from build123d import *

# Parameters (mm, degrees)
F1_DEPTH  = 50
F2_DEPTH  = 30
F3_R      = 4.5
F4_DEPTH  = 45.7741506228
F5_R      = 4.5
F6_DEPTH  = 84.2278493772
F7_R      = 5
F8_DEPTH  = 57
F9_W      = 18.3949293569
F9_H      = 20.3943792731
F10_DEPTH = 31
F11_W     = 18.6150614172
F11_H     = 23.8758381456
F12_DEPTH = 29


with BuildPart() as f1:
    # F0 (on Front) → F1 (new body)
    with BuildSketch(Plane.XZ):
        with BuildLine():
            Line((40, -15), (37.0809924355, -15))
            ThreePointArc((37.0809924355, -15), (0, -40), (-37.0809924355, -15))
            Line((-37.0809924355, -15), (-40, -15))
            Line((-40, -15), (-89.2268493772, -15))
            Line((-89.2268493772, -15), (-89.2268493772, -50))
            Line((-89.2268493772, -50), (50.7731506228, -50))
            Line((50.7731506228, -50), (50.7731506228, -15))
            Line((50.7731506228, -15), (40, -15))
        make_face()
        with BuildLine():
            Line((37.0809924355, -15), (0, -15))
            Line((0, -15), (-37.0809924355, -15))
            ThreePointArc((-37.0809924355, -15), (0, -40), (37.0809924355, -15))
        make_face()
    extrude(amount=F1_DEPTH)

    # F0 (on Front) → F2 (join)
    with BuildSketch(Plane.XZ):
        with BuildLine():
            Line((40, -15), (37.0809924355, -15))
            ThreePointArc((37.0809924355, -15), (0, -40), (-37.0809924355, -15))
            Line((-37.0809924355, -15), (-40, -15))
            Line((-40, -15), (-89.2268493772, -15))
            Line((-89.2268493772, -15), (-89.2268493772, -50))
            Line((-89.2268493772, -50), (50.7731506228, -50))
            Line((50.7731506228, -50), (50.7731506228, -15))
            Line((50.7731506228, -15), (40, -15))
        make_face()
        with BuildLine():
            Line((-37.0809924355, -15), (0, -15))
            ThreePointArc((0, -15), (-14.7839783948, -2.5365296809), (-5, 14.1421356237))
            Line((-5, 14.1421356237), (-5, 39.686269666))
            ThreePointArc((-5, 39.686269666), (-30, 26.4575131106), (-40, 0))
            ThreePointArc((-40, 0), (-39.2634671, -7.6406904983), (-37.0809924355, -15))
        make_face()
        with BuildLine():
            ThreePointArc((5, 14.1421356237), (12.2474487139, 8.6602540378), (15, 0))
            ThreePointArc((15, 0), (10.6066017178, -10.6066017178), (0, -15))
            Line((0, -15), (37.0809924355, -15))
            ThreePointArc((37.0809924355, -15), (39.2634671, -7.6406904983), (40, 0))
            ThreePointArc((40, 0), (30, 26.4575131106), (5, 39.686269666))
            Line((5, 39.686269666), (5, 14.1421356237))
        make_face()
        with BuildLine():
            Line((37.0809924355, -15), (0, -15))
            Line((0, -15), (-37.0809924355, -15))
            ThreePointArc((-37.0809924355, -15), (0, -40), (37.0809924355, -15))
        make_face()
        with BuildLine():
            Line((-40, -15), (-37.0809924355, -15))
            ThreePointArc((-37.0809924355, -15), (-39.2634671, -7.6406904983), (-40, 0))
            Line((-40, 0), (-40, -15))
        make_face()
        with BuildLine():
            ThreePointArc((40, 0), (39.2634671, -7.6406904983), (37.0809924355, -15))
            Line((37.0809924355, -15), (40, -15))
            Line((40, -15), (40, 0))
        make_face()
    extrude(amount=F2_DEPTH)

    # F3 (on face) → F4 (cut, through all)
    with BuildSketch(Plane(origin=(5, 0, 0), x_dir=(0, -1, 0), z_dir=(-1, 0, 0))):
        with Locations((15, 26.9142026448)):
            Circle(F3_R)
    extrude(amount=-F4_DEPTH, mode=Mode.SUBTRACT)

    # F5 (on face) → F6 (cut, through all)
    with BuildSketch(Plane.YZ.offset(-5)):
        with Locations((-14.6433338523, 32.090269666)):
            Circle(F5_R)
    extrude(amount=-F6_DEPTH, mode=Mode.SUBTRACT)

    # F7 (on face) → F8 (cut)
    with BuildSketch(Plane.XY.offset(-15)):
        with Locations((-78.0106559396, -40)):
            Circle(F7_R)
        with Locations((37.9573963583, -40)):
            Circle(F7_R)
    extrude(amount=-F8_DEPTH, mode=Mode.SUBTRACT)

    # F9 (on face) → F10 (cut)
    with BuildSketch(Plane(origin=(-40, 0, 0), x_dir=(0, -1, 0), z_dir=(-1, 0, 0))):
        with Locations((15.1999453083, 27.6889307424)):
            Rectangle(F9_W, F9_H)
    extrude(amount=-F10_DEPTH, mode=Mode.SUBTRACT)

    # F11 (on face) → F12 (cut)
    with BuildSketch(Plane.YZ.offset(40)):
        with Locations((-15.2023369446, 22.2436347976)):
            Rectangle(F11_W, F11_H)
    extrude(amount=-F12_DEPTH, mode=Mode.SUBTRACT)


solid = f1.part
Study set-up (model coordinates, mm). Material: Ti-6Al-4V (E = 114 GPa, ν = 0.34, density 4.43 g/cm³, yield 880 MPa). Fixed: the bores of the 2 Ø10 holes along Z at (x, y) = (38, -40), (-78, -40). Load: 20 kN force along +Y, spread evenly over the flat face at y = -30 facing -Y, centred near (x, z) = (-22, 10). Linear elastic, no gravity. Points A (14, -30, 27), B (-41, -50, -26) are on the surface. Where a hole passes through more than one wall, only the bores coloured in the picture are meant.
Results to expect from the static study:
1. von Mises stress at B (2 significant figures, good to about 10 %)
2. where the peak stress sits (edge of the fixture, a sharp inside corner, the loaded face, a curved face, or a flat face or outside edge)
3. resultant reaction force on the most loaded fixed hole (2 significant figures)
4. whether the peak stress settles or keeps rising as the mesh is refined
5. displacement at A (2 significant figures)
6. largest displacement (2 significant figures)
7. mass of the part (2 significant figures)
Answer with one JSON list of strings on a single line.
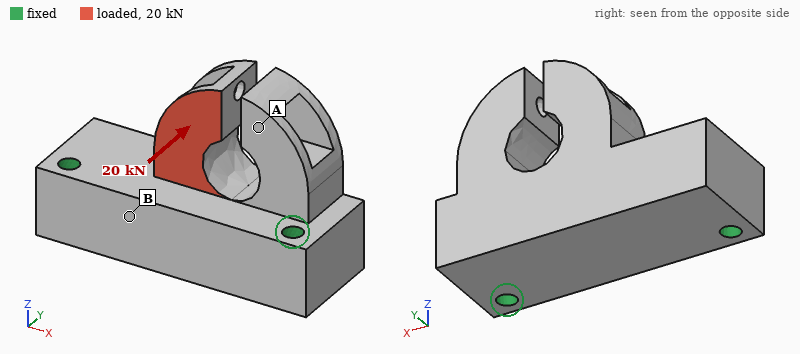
["37 MPa", "edge of the fixture", "14 kN", "keeps rising", "0.048 mm", "0.28 mm", "1.4 kg"]
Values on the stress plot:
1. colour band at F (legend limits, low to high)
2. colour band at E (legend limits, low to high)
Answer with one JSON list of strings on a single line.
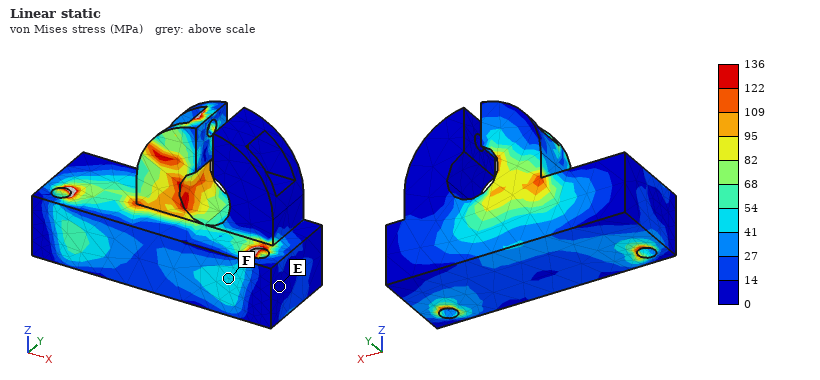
["41 to 54 MPa", "0 to 14 MPa"]
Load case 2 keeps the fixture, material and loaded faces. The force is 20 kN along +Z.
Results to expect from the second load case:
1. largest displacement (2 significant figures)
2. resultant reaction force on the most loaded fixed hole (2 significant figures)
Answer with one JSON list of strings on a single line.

["0.12 mm", "11 kN"]
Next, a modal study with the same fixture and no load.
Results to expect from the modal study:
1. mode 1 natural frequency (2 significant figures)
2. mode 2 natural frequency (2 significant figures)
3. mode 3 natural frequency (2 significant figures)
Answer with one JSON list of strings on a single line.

["4000 Hz", "5400 Hz", "5700 Hz"]
